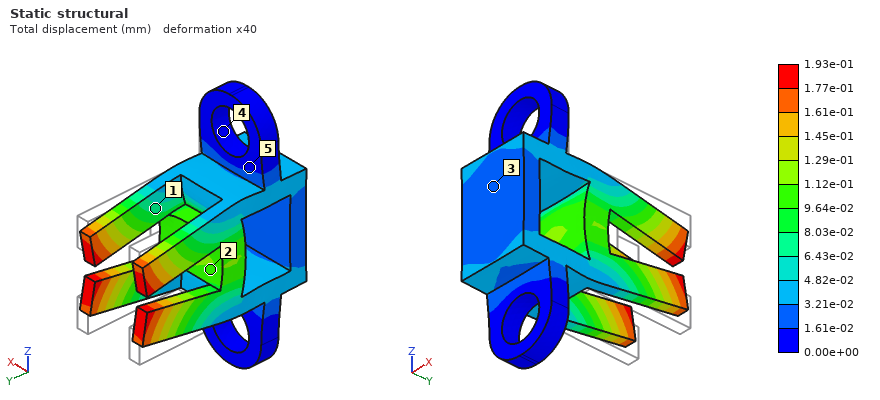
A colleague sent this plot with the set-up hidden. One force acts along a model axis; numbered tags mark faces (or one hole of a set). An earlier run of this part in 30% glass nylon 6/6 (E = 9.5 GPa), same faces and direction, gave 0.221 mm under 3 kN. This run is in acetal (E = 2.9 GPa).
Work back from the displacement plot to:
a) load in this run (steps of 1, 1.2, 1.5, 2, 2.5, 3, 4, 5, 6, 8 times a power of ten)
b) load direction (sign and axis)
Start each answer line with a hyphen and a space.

- 800 N
- -Y
